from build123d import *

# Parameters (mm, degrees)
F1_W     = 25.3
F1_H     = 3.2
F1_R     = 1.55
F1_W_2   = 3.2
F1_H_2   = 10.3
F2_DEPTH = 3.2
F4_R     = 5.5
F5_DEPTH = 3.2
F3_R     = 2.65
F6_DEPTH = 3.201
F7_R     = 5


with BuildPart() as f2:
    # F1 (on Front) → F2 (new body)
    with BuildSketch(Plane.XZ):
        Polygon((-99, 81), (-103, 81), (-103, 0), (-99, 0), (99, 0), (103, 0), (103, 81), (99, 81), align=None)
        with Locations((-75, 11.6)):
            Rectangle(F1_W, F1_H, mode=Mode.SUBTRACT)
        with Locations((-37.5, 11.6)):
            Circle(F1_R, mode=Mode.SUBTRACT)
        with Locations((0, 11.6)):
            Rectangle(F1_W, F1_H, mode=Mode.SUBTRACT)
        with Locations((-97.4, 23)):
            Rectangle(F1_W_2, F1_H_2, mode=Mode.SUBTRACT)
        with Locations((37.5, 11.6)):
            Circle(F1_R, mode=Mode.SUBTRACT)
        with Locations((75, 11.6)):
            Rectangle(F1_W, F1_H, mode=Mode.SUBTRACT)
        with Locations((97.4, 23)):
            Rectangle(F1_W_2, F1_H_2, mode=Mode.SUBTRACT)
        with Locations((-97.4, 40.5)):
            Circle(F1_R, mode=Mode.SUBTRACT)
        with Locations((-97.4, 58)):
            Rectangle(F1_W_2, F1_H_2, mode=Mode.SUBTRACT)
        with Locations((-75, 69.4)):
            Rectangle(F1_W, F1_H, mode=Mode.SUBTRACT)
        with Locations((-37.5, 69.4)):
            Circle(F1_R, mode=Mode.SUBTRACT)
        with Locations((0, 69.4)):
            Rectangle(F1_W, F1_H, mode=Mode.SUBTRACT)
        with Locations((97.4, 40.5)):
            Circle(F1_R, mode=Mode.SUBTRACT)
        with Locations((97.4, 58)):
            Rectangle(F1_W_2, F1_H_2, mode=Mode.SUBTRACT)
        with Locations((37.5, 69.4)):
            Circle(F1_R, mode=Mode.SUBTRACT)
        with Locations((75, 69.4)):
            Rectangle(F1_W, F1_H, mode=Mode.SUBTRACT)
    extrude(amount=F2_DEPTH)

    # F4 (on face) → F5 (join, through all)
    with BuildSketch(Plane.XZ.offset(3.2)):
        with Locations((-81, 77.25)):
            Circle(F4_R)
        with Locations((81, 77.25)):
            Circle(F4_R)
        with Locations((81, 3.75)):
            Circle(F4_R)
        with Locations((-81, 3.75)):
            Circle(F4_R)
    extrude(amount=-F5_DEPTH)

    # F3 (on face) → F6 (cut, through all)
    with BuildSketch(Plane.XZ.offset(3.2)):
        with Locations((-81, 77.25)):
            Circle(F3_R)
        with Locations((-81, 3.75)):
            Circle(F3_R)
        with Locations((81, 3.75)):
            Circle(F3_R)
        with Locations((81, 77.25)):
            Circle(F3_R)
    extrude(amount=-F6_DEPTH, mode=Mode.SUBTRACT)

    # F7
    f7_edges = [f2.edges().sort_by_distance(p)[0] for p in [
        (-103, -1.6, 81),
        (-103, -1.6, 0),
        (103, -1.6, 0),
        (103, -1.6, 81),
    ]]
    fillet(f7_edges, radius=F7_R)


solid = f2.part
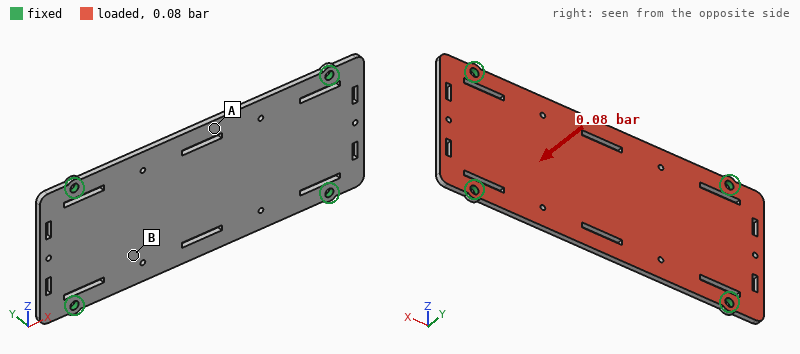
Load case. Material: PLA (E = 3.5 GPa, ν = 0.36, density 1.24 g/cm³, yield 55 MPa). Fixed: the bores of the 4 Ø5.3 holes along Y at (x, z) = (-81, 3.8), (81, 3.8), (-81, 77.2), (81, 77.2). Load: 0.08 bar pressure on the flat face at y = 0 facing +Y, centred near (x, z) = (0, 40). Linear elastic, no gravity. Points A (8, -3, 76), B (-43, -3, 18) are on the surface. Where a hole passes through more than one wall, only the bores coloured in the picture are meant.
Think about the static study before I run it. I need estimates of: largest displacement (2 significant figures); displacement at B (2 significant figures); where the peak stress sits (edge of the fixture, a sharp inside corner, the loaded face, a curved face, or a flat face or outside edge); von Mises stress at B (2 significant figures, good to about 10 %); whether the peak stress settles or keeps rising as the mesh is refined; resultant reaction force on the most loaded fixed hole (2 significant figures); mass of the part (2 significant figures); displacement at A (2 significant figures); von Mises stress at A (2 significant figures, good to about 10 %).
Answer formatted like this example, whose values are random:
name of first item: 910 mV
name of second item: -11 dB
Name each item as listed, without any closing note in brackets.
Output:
largest displacement: 2.3 mm
displacement at B: 1.3 mm
where the peak stress sits: edge of the fixture
von Mises stress at B: 2.8 MPa
whether the peak stress settles or keeps rising as the mesh is refined: keeps rising
resultant reaction force on the most loaded fixed hole: 32 N
mass of the part: 63 g
displacement at A: 2.2 mm
von Mises stress at A: 6.9 MPa
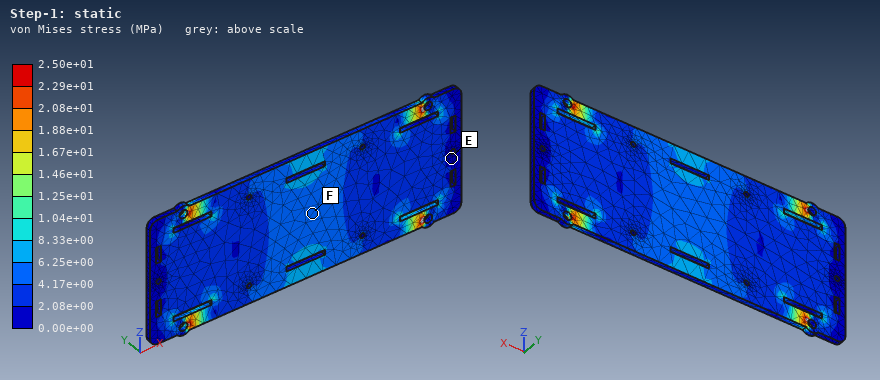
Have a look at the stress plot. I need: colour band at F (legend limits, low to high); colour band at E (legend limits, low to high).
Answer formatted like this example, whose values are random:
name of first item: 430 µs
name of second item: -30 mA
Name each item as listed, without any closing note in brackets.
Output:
colour band at F: 4.17e+00 to 6.25e+00 MPa
colour band at E: 0.00e+00 to 2.08e+00 MPa
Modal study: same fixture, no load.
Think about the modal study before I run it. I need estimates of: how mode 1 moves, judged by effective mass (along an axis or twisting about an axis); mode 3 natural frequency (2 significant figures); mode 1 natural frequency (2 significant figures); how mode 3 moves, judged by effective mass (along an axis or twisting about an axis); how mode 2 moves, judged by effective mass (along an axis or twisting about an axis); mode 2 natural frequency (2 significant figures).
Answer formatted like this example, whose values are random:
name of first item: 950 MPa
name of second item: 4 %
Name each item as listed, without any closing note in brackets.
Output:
how mode 1 moves, judged by effective mass: along Y
mode 3 natural frequency: 470 Hz
mode 1 natural frequency: 170 Hz
how mode 3 moves, judged by effective mass: twisting about Z
how mode 2 moves, judged by effective mass: twisting about X
mode 2 natural frequency: 340 Hz
